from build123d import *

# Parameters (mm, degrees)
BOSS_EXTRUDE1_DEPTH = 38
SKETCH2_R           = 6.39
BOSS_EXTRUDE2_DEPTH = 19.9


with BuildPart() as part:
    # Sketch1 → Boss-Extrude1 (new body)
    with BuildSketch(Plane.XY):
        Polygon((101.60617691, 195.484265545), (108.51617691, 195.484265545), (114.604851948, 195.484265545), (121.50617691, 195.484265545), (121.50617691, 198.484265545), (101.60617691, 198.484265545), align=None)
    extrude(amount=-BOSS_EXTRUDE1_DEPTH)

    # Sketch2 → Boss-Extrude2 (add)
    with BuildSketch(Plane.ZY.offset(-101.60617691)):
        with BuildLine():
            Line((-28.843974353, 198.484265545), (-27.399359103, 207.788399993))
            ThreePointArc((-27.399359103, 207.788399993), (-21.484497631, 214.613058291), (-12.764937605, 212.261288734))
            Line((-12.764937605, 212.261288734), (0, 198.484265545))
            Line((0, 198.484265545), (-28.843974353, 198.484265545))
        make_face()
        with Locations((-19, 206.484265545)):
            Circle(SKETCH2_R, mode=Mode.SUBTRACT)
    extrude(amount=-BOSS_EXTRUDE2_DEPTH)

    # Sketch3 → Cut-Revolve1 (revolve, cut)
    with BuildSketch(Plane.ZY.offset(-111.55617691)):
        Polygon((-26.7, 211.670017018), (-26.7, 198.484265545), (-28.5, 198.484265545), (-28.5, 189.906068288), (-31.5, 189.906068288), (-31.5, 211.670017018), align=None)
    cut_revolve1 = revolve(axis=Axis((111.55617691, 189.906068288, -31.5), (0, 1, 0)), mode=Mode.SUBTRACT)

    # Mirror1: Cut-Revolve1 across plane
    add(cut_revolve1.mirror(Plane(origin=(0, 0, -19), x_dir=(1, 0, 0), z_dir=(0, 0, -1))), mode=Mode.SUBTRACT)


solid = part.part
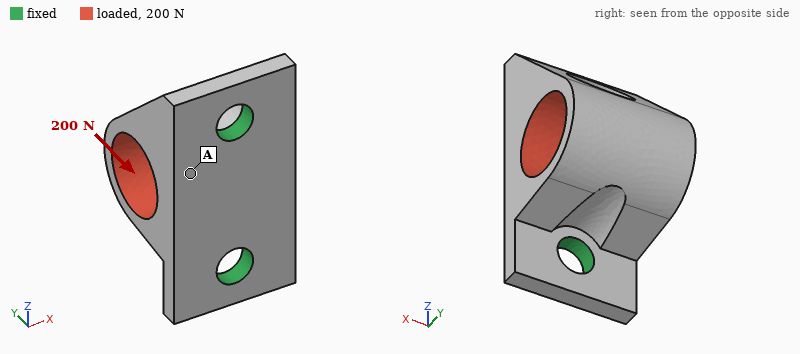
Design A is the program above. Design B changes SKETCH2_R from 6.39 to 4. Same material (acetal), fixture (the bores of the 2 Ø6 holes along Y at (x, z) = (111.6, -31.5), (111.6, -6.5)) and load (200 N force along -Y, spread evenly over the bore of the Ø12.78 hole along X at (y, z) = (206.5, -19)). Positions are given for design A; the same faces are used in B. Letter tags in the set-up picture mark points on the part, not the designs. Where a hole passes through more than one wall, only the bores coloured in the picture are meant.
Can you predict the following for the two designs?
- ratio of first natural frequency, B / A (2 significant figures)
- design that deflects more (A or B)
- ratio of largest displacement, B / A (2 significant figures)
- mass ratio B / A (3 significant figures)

0.84
A
0.68
1.29
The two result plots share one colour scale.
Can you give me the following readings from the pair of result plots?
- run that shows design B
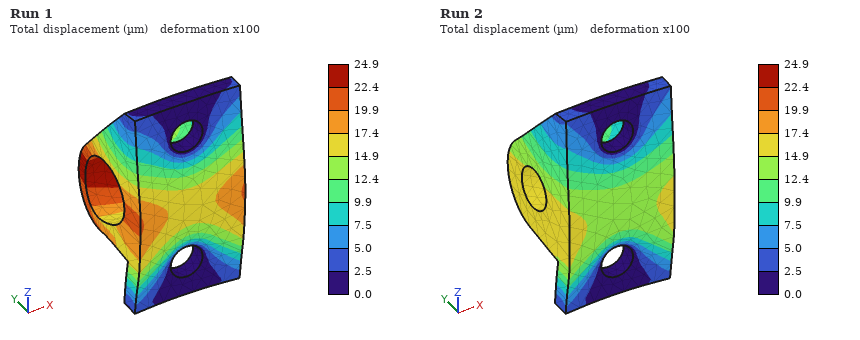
Run 2
